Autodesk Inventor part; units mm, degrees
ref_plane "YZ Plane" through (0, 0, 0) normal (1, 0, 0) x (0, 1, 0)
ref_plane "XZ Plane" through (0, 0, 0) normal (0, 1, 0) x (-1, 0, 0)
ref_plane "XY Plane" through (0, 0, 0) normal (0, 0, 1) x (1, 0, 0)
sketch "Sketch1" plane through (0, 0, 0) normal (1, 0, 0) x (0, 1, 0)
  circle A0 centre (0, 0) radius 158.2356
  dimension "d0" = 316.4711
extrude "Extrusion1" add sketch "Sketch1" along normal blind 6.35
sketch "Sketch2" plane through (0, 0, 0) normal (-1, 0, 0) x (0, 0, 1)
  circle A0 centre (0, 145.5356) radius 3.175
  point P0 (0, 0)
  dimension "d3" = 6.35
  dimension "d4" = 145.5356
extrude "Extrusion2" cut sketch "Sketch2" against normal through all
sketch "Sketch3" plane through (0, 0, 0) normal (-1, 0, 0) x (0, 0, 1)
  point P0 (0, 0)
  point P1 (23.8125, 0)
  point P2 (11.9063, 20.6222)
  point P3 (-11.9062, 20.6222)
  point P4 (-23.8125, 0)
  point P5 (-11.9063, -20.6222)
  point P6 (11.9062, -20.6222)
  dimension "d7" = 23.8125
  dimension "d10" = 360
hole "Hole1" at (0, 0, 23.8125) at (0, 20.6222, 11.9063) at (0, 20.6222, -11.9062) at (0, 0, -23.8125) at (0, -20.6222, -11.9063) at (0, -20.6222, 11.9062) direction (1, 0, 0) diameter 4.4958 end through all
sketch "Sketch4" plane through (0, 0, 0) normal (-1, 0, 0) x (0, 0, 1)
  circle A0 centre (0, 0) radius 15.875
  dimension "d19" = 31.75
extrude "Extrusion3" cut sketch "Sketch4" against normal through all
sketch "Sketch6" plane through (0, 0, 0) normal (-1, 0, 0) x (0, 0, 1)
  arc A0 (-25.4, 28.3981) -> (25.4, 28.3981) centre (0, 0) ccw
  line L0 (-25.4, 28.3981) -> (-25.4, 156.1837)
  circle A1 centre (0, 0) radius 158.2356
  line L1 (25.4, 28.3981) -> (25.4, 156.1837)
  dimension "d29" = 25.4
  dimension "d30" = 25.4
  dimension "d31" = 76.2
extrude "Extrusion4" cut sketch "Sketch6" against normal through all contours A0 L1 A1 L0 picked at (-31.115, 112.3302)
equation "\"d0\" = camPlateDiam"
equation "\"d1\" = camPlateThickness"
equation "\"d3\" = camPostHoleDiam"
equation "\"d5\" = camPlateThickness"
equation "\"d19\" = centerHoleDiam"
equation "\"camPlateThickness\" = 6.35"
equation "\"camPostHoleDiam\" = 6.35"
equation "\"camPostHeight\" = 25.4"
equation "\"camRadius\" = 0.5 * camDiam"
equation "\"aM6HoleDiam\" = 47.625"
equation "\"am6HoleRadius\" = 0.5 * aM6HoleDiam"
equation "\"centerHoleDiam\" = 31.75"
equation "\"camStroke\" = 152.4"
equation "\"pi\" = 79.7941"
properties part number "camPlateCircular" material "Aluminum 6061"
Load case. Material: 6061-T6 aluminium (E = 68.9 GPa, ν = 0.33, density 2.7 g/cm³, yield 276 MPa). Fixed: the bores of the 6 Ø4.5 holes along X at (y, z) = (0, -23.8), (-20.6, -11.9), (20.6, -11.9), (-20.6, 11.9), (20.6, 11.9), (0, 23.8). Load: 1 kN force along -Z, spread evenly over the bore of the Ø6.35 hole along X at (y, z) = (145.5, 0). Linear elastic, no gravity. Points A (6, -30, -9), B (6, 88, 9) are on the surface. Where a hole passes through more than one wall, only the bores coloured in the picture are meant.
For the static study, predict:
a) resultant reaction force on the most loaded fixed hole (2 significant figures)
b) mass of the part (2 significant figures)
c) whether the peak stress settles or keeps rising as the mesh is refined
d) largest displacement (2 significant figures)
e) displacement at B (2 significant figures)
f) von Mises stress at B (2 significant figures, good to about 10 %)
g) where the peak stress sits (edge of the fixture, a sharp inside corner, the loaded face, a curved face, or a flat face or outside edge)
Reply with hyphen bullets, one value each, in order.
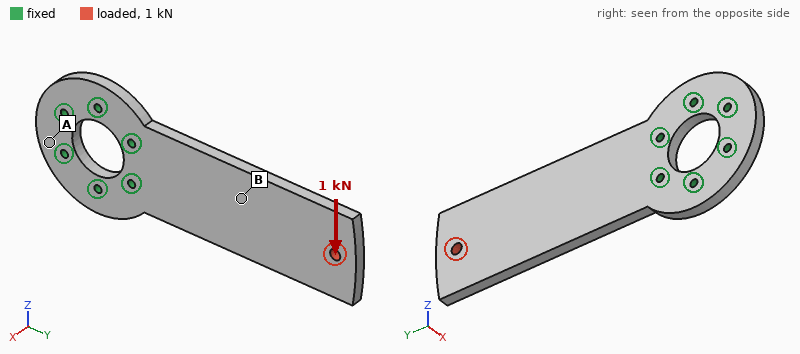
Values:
- 2.4 kN
- 170 g
- keeps rising
- 0.19 mm
- 0.064 mm
- 10 MPa
- edge of the fixture
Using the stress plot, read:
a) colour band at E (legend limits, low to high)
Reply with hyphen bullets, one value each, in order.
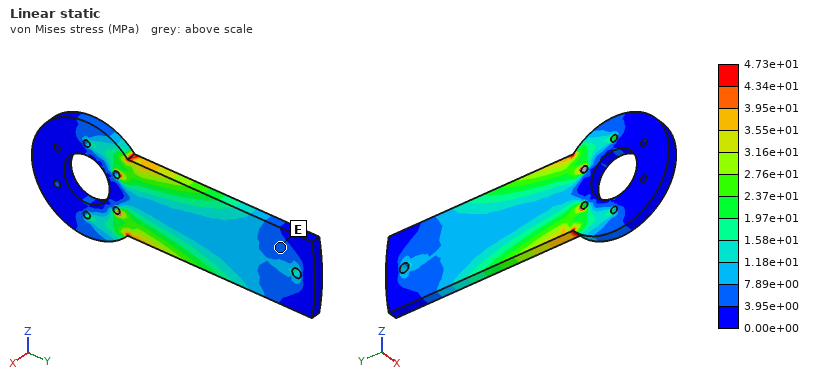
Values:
- 3.95e+00 to 7.89e+00 MPa
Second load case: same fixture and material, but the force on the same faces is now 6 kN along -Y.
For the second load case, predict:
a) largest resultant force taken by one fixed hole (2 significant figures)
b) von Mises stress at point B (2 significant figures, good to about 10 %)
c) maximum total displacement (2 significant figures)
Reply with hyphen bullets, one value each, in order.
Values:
- 2.4 kN
- 19 MPa
- 45 µm
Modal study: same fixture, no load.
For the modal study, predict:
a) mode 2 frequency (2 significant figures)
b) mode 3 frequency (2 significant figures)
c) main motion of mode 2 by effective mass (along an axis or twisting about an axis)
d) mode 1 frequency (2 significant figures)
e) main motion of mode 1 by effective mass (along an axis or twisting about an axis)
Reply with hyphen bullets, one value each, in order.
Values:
- 1500 Hz
- 1700 Hz
- twisting about Y
- 280 Hz
- along X
